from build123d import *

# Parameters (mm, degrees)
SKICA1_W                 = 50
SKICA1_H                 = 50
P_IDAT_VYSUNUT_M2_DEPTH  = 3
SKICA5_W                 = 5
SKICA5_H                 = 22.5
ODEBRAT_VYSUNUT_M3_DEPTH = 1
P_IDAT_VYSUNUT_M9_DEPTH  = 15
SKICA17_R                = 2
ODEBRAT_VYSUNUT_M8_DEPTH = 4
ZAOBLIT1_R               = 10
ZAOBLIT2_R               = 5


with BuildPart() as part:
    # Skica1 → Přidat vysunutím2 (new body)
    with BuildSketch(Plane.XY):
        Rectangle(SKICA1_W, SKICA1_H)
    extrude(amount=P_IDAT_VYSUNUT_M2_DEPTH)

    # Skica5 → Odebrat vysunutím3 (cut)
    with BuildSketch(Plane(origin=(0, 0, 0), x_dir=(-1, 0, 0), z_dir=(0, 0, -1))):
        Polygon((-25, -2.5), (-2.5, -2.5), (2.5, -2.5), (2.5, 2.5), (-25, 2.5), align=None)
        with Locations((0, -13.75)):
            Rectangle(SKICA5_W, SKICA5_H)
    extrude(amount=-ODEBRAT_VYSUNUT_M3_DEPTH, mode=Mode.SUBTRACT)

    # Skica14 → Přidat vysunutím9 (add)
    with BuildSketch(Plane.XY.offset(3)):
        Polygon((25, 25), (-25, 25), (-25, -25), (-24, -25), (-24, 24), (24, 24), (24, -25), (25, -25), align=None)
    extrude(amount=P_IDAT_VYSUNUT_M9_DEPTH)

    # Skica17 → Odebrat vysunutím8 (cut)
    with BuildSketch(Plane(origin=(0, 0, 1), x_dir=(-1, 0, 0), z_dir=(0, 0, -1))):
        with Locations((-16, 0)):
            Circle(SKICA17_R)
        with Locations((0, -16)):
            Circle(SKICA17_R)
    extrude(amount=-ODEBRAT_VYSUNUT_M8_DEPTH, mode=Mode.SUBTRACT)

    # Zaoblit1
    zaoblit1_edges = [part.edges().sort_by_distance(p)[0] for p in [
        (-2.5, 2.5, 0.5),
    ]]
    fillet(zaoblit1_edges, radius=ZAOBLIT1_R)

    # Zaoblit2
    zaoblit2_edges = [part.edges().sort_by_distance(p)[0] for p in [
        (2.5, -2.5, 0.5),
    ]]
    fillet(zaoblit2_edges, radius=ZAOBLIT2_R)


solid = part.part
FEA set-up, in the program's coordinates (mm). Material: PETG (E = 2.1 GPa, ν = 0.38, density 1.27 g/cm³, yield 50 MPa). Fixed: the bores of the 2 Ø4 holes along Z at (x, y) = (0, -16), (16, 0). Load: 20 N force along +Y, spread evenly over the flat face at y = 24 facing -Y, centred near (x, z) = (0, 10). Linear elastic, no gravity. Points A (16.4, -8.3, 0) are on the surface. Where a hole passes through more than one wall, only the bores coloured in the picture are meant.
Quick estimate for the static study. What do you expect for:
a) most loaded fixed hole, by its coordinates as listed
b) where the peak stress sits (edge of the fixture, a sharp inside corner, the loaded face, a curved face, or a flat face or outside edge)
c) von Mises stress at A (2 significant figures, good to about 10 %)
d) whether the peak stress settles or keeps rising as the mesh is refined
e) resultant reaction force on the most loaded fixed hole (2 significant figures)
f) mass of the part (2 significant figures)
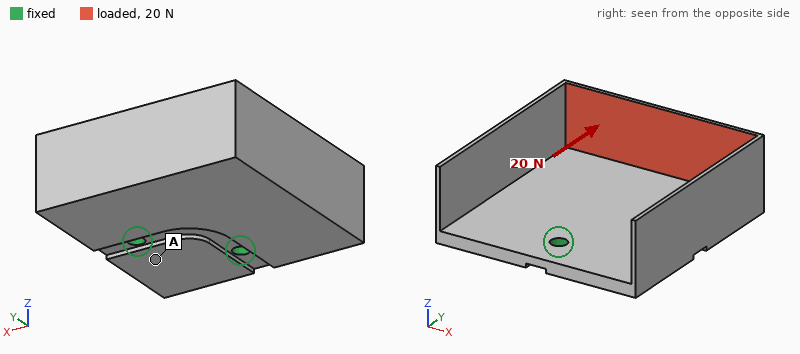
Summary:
(0, -16)
edge of the fixture
0.92 MPa
keeps rising
14 N
12 g
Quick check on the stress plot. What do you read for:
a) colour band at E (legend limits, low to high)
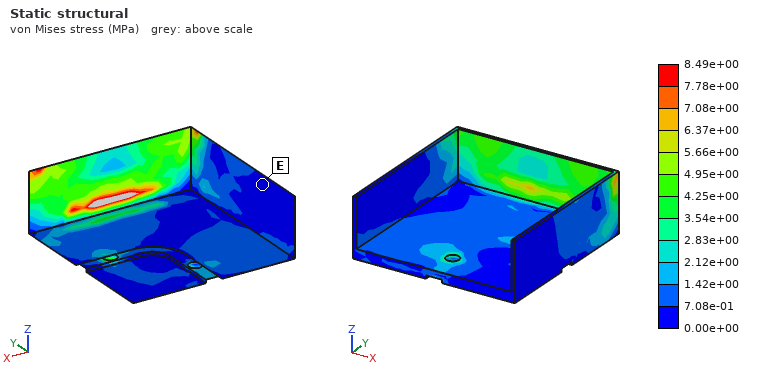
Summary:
0.00e+00 to 7.08e-01 MPa
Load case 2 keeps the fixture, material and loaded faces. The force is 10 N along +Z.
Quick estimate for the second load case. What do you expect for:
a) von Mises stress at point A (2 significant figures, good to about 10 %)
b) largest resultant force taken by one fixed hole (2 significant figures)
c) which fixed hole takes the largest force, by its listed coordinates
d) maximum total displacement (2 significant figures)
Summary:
1.0 MPa
10 N
(16, 0)
0.87 mm
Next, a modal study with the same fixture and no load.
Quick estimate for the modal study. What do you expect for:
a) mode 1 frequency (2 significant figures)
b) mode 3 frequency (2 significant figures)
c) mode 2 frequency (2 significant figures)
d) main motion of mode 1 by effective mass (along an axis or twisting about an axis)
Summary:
300 Hz
830 Hz
670 Hz
along Z
